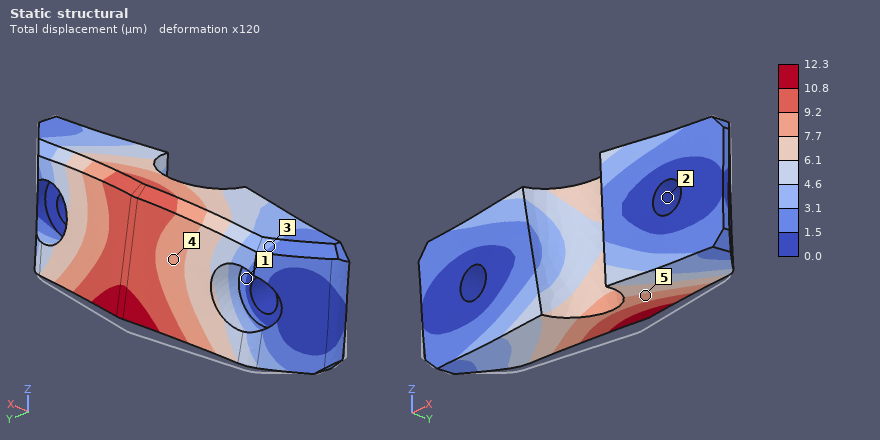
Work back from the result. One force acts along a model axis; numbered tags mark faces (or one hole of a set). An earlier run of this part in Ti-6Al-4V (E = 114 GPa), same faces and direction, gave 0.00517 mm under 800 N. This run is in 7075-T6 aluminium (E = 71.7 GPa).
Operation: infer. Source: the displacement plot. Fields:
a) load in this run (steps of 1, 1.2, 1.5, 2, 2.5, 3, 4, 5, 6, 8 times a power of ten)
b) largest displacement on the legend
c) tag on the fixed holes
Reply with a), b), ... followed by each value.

a) 1.2 kN
b) 12.3 µm
c) 2
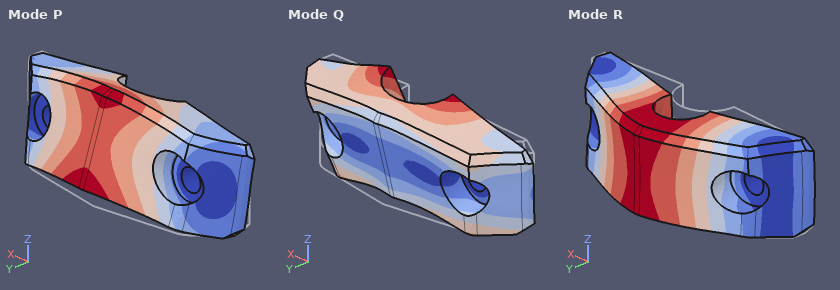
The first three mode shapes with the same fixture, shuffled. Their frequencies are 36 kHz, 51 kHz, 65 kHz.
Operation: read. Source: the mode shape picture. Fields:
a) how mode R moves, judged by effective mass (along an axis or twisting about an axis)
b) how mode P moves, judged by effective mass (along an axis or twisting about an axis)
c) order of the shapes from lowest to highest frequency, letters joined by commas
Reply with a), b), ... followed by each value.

a) along Y
b) along Z
c) P, R, Q
